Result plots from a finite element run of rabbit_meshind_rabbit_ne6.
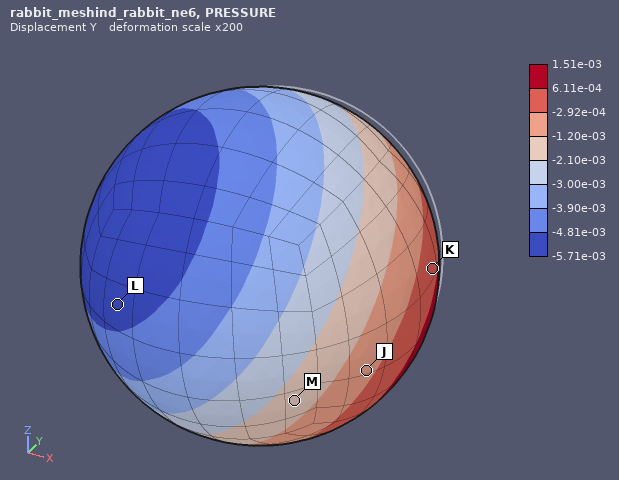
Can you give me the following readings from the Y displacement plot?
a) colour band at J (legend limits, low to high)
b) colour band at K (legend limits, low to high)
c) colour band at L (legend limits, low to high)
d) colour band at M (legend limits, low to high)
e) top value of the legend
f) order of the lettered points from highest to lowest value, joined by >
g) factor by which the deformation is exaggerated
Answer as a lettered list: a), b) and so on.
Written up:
a) -1.20e-03 to -2.92e-04
b) -2.92e-04 to 6.11e-04
c) -5.71e-03 to -4.81e-03
d) -2.10e-03 to -1.20e-03
e) 1.51e-03
f) K > J > M > L
g) 200
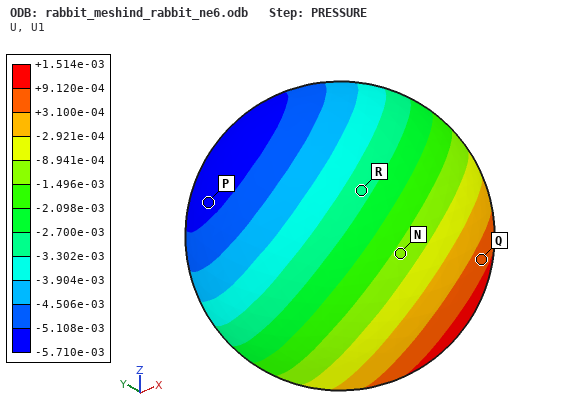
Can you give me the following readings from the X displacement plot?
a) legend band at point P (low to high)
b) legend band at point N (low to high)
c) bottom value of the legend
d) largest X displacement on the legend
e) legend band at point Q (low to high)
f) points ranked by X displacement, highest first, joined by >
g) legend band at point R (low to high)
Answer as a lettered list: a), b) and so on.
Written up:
a) -5.710e-03 to -5.108e-03
b) -1.496e-03 to -8.941e-04
c) -5.710e-03
d) +1.514e-03
e) +3.100e-04 to +9.120e-04
f) Q > N > R > P
g) -3.302e-03 to -2.700e-03
